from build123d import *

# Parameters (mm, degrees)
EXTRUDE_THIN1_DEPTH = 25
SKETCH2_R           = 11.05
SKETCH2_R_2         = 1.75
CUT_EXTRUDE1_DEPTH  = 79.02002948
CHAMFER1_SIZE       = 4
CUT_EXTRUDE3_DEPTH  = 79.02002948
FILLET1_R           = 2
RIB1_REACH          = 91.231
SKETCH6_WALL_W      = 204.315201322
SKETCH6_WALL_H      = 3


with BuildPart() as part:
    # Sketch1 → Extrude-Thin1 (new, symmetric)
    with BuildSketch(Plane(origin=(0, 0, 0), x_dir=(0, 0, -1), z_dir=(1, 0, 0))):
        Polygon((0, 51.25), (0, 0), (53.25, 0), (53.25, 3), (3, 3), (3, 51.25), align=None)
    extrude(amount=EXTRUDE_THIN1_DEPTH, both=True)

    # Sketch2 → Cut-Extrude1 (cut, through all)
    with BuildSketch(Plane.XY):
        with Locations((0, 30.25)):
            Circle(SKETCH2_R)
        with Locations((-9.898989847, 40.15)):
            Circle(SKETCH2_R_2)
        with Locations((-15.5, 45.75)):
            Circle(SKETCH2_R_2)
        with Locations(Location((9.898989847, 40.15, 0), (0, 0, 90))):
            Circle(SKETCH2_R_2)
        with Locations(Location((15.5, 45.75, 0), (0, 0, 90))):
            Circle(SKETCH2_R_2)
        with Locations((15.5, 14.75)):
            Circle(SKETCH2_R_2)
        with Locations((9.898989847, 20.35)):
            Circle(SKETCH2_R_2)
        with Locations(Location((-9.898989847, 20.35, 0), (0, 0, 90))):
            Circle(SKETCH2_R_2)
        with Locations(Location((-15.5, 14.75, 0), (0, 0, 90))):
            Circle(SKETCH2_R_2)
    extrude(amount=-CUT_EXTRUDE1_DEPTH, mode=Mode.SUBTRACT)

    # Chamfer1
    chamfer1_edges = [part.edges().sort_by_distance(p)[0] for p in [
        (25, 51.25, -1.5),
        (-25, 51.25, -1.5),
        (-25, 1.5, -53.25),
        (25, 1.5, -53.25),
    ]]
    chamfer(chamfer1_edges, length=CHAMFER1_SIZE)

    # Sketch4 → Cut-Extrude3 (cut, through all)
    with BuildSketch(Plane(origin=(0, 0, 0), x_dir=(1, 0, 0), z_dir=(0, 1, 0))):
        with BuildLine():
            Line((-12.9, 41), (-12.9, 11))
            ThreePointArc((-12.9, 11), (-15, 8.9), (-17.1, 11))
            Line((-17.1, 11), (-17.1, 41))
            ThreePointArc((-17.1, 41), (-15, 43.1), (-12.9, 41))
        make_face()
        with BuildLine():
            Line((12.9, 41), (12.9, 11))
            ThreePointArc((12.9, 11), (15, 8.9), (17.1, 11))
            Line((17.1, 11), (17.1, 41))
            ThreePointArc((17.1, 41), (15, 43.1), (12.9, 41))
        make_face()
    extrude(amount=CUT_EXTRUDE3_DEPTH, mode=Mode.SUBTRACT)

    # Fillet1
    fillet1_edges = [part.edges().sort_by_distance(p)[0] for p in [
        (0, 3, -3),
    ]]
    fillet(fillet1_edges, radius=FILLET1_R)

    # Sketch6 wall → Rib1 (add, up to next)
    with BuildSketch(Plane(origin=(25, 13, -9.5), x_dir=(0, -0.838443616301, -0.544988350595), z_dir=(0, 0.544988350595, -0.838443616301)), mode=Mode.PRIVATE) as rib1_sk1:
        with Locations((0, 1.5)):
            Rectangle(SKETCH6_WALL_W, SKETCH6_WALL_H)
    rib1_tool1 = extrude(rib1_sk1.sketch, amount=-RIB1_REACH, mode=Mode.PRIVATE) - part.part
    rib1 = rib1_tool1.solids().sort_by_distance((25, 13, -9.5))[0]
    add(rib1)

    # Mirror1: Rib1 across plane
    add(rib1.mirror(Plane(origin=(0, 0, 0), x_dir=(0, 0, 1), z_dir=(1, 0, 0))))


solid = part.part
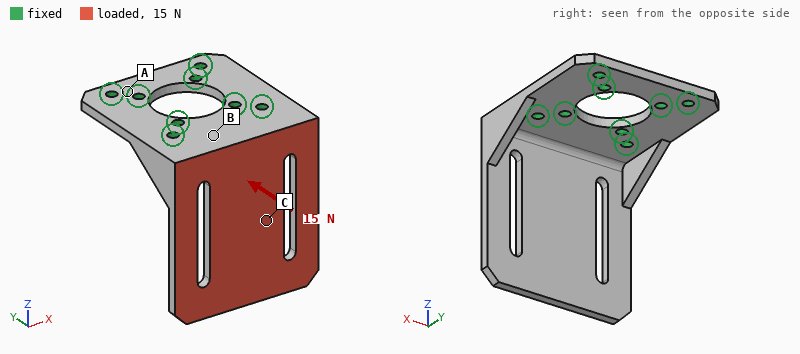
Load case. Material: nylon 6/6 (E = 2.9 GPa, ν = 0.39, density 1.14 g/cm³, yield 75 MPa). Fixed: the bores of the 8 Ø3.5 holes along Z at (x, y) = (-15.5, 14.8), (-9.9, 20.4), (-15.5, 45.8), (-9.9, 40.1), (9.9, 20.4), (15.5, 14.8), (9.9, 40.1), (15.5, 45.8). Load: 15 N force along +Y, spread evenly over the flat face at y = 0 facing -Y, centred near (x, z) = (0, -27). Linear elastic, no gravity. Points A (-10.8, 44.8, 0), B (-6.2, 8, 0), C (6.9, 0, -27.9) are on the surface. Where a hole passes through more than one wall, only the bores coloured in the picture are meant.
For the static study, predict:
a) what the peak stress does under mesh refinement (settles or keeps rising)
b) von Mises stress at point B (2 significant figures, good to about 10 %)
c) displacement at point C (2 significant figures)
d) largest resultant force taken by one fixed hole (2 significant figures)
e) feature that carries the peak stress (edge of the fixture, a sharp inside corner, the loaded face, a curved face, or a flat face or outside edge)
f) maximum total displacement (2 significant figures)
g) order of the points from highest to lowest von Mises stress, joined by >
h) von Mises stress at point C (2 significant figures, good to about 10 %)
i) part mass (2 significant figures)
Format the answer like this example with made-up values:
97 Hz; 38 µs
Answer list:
keeps rising; 1.9 MPa; 0.33 mm; 10 N; edge of the fixture; 0.81 mm; B > C > A; 1.1 MPa; 16 g
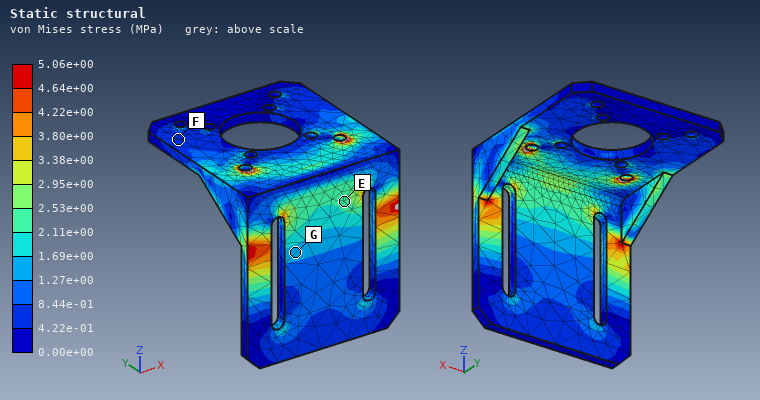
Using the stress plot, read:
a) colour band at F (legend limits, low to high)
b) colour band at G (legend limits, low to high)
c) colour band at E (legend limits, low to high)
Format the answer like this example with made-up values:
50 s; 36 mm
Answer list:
4.22e-01 to 8.44e-01 MPa; 1.27e+00 to 1.69e+00 MPa; 2.11e+00 to 2.53e+00 MPa
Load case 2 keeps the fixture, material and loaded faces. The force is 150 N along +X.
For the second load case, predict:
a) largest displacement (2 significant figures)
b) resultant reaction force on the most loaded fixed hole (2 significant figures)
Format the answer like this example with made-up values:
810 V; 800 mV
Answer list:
0.94 mm; 150 N
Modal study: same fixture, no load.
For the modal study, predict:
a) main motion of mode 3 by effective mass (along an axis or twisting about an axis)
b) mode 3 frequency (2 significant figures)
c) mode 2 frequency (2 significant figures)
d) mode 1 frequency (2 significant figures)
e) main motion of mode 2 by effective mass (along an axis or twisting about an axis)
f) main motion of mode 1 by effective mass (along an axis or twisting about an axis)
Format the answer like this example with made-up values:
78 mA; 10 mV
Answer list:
along X; 1000 Hz; 670 Hz; 300 Hz; along X; along Y
